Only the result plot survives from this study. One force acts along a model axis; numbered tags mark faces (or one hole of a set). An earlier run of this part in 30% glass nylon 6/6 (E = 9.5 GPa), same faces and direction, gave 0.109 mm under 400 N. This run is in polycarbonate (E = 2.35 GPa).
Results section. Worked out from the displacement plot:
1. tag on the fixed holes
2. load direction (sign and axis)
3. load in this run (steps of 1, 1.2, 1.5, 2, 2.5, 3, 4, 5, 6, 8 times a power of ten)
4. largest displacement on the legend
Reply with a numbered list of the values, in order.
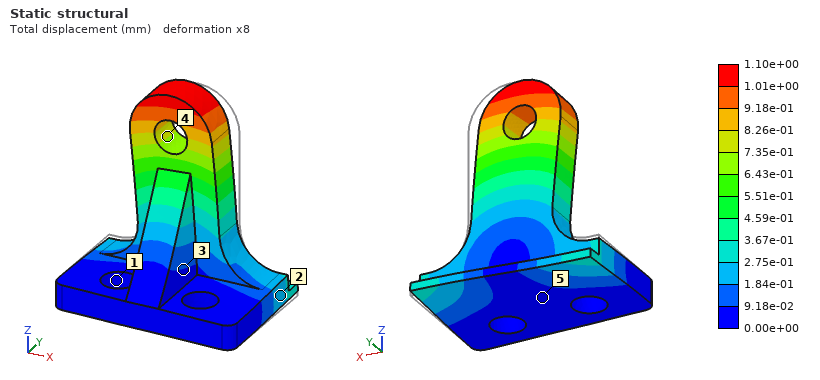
1. 1
2. -X
3. 1 kN
4. 1.10e+00 mm
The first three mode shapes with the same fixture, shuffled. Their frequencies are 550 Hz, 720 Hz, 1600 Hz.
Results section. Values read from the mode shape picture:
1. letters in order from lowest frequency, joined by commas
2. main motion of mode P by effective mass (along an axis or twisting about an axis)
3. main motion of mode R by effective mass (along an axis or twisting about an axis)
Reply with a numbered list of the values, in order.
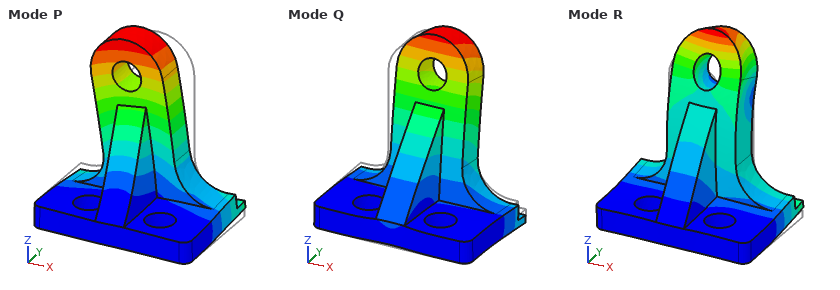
1. Q, P, R
2. along X
3. along Z
